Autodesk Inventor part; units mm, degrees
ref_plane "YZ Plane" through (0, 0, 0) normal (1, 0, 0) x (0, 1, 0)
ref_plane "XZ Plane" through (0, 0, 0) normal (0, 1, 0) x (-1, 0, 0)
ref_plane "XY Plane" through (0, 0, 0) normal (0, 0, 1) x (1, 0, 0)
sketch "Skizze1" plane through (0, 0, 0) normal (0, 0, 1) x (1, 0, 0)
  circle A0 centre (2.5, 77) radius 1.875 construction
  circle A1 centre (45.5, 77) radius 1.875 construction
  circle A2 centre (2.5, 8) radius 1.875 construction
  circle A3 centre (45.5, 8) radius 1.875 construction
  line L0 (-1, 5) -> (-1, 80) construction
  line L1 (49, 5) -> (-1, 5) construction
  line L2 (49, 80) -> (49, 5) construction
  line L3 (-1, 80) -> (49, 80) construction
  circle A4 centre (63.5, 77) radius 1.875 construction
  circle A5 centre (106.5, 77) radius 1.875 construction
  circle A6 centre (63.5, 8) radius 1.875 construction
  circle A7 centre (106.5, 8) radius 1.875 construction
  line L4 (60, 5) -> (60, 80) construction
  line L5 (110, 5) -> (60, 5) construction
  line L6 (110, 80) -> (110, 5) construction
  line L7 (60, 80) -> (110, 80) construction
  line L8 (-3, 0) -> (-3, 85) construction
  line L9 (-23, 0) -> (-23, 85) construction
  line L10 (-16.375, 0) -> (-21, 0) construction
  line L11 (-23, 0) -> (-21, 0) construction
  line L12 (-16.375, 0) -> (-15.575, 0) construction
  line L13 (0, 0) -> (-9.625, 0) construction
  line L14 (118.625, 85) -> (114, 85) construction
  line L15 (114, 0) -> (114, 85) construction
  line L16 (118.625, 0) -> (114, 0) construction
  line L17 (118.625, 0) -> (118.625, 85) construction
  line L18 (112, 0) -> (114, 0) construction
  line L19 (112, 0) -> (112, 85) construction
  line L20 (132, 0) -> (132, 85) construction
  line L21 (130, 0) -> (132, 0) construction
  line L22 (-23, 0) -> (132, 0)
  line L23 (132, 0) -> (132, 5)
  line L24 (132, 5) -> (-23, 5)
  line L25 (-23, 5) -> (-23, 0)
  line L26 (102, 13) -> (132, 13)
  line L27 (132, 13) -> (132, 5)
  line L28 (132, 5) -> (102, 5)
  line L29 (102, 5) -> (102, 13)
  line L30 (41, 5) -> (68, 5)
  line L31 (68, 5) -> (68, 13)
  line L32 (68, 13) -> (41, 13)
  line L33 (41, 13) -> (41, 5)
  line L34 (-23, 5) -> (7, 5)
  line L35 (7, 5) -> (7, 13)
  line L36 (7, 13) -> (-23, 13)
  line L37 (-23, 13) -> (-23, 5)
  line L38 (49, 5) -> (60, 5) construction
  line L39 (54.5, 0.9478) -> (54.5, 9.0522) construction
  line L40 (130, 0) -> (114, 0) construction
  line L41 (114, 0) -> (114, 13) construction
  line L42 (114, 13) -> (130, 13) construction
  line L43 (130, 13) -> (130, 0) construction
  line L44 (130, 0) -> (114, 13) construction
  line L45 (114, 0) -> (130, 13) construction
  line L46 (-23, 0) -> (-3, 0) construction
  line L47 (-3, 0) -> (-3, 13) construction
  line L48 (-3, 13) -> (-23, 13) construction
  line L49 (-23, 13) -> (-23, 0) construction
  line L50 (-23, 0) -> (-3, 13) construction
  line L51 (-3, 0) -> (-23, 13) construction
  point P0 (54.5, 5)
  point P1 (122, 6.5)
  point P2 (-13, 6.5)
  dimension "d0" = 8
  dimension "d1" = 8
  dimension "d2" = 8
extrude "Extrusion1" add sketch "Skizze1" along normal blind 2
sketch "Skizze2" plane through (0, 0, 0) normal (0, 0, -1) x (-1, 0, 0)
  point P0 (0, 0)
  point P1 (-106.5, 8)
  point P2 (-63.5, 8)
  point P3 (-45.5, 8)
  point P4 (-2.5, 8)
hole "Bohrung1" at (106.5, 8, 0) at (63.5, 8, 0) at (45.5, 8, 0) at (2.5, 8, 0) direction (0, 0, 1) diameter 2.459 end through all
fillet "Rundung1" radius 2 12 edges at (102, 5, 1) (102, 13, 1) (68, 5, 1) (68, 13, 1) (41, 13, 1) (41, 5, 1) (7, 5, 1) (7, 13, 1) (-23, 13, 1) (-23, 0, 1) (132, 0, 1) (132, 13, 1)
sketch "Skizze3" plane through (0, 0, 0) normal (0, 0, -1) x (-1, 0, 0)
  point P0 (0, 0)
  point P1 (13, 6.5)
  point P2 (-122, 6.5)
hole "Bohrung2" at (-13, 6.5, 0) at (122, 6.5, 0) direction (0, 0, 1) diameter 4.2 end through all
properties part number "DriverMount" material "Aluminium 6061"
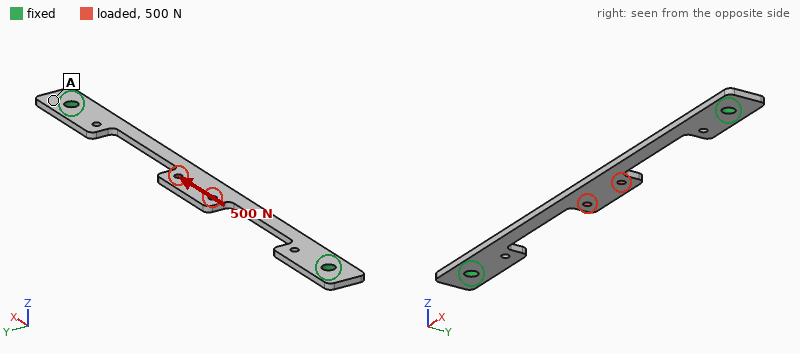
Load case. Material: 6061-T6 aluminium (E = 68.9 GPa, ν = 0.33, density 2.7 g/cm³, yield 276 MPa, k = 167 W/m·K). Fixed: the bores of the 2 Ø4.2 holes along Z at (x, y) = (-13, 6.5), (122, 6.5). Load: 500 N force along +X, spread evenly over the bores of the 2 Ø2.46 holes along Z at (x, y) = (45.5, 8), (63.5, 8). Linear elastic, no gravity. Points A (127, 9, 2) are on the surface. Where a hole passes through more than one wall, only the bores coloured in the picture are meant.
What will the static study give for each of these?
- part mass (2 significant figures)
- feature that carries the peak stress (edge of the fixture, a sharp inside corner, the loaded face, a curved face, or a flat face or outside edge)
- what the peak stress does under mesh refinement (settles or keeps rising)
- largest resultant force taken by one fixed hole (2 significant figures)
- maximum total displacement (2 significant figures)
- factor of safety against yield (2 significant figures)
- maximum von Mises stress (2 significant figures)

7.7 g
a curved face
settles
250 N
0.10 mm
1.6
180 MPa
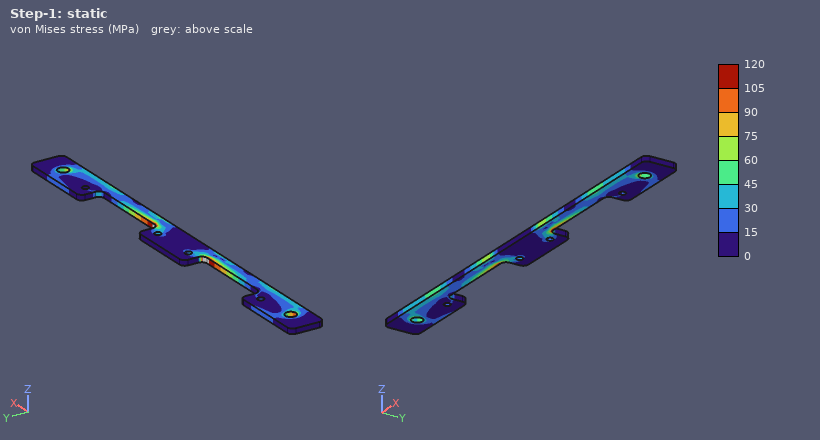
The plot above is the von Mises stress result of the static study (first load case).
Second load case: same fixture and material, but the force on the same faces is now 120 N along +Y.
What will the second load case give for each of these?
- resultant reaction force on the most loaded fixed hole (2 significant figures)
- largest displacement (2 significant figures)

77 N
0.26 mm
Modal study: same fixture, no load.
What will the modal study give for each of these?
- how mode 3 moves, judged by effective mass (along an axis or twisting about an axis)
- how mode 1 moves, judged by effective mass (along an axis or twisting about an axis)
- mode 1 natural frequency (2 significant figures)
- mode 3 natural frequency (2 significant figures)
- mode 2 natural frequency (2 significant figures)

along Y
along Z
610 Hz
2100 Hz
1800 Hz
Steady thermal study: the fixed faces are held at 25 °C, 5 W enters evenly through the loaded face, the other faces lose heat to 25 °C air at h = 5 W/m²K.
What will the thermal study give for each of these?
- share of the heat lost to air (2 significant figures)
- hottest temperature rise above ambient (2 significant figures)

9.4 %
67 K
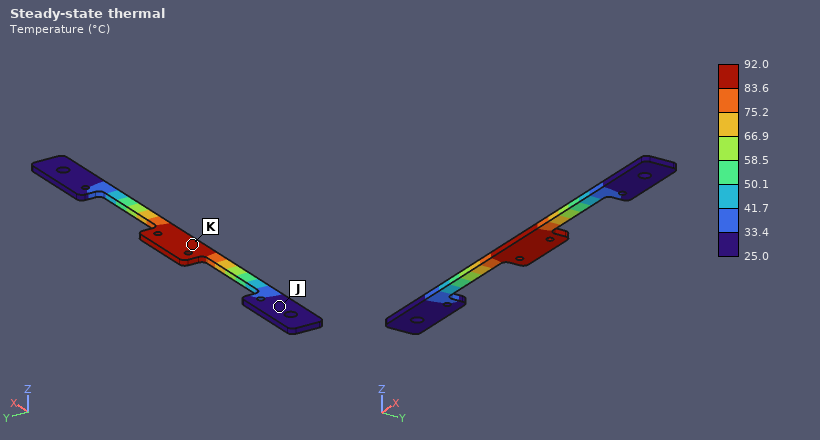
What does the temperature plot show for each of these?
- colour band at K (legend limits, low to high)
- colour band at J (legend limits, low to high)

83.6 to 92.0 °C
25.0 to 33.4 °C
